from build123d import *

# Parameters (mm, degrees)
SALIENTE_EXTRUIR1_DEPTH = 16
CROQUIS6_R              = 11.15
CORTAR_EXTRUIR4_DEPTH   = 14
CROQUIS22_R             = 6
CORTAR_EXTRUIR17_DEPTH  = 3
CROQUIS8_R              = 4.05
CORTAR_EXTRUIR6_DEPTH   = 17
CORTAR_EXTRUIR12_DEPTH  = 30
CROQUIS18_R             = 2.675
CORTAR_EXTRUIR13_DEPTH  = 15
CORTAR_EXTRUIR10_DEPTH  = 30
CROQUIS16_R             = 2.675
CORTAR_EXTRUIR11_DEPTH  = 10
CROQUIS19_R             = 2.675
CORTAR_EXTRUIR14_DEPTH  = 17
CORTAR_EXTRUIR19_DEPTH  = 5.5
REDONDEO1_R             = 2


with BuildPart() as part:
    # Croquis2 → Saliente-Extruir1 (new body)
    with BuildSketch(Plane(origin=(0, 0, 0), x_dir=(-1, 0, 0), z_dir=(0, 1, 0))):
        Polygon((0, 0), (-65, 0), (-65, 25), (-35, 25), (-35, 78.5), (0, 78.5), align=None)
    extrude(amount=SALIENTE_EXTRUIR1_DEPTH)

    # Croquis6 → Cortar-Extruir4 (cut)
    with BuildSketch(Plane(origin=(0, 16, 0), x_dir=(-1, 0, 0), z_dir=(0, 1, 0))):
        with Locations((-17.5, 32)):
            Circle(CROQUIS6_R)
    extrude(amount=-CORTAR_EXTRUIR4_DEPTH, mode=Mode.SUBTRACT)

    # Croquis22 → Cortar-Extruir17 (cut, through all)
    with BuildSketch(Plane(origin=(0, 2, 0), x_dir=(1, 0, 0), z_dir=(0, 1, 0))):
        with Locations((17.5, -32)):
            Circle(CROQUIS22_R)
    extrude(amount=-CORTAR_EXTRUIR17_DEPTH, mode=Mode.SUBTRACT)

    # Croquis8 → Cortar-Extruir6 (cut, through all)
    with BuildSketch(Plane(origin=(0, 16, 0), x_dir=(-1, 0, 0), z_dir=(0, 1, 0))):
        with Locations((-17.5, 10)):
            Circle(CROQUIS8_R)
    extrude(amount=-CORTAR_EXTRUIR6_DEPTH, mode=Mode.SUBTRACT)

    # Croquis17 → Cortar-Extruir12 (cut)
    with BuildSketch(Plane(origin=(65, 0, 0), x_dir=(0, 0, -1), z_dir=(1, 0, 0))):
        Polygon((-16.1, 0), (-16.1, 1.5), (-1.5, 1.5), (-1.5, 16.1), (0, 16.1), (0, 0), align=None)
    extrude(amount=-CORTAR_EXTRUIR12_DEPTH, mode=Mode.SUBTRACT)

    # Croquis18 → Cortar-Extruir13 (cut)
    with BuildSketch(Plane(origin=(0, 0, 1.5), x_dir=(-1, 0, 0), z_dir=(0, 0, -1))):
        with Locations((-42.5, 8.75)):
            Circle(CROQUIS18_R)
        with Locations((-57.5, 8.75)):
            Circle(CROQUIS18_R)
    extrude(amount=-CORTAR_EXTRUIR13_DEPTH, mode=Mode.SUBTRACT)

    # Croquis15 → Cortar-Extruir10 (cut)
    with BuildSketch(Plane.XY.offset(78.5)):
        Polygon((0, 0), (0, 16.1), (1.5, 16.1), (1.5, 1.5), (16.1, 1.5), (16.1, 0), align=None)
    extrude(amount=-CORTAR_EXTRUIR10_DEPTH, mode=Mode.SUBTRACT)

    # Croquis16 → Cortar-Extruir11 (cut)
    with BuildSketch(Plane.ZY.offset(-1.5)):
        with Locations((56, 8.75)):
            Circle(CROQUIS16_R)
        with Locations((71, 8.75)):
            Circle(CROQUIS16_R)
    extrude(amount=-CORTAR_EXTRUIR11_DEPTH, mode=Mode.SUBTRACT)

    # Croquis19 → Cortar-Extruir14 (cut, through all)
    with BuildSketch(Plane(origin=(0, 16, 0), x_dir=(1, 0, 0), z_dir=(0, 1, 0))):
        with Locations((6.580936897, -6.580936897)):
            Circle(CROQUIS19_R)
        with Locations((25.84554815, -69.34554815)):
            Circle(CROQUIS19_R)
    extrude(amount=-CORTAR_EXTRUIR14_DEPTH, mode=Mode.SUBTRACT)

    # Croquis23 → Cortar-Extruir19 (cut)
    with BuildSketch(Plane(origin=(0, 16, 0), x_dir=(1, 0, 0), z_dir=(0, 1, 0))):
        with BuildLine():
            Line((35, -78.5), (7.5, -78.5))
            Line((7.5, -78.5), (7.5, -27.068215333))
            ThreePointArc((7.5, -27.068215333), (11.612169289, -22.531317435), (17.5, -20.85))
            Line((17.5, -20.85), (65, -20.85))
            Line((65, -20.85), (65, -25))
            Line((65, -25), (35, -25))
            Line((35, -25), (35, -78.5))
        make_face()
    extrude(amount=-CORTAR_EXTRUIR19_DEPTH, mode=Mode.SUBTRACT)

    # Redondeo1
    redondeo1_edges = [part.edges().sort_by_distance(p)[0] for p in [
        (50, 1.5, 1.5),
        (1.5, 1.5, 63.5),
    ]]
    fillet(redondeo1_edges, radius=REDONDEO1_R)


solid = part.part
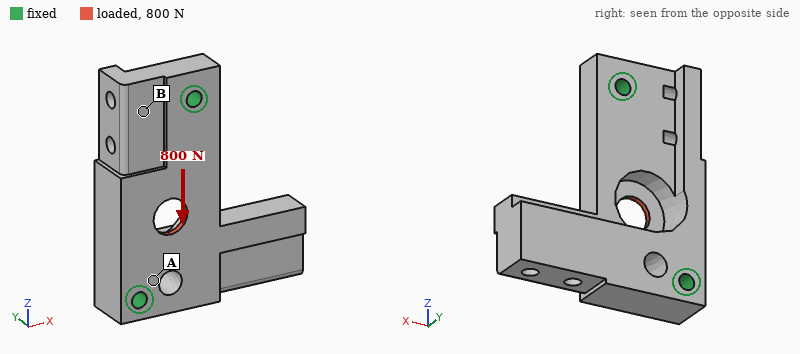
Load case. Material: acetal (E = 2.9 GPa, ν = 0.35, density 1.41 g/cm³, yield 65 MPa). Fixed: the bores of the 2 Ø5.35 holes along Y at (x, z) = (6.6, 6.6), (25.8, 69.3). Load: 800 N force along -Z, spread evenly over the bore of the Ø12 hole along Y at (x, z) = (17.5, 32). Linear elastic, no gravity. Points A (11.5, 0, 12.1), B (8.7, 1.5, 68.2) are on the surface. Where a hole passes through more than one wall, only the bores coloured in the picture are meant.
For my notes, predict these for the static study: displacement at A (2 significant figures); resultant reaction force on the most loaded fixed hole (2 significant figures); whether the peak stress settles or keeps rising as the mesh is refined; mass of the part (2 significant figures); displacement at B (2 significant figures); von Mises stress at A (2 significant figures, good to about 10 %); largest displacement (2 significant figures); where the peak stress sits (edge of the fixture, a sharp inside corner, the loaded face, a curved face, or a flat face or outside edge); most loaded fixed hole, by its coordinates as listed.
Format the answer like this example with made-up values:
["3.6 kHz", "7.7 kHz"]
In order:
["12 µm", "430 N", "keeps rising", "53 g", "21 µm", "3.4 MPa", "74 µm", "a sharp inside corner", "(6.6, 6.6)"]
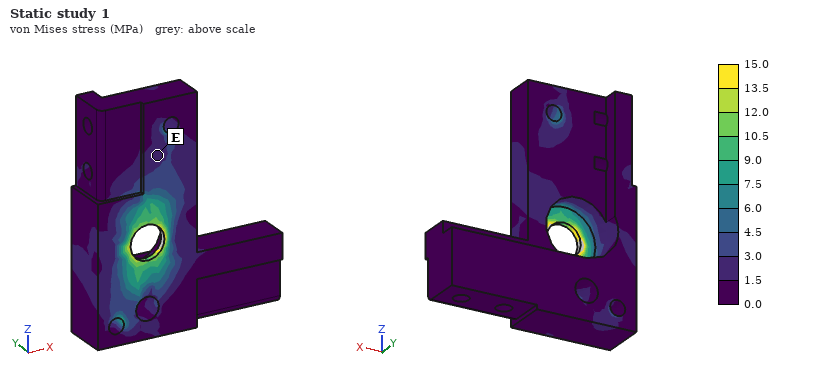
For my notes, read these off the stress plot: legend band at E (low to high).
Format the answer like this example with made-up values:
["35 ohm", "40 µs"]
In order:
["1.5 to 3.0 MPa"]
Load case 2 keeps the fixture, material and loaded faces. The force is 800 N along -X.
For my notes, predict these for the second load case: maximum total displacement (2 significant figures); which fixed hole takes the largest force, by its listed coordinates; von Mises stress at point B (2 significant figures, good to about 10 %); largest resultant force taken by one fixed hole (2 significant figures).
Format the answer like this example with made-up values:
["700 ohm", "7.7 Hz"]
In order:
["0.20 mm", "(6.6, 6.6)", "1.3 MPa", "470 N"]
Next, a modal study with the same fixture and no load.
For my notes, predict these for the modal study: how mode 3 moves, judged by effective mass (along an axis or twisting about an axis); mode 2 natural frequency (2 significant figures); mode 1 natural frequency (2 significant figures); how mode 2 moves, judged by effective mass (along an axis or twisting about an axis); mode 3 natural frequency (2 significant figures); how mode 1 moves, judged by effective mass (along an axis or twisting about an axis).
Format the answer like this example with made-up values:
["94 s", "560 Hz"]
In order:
["along Y", "1900 Hz", "950 Hz", "along Z", "2800 Hz", "along Y"]
